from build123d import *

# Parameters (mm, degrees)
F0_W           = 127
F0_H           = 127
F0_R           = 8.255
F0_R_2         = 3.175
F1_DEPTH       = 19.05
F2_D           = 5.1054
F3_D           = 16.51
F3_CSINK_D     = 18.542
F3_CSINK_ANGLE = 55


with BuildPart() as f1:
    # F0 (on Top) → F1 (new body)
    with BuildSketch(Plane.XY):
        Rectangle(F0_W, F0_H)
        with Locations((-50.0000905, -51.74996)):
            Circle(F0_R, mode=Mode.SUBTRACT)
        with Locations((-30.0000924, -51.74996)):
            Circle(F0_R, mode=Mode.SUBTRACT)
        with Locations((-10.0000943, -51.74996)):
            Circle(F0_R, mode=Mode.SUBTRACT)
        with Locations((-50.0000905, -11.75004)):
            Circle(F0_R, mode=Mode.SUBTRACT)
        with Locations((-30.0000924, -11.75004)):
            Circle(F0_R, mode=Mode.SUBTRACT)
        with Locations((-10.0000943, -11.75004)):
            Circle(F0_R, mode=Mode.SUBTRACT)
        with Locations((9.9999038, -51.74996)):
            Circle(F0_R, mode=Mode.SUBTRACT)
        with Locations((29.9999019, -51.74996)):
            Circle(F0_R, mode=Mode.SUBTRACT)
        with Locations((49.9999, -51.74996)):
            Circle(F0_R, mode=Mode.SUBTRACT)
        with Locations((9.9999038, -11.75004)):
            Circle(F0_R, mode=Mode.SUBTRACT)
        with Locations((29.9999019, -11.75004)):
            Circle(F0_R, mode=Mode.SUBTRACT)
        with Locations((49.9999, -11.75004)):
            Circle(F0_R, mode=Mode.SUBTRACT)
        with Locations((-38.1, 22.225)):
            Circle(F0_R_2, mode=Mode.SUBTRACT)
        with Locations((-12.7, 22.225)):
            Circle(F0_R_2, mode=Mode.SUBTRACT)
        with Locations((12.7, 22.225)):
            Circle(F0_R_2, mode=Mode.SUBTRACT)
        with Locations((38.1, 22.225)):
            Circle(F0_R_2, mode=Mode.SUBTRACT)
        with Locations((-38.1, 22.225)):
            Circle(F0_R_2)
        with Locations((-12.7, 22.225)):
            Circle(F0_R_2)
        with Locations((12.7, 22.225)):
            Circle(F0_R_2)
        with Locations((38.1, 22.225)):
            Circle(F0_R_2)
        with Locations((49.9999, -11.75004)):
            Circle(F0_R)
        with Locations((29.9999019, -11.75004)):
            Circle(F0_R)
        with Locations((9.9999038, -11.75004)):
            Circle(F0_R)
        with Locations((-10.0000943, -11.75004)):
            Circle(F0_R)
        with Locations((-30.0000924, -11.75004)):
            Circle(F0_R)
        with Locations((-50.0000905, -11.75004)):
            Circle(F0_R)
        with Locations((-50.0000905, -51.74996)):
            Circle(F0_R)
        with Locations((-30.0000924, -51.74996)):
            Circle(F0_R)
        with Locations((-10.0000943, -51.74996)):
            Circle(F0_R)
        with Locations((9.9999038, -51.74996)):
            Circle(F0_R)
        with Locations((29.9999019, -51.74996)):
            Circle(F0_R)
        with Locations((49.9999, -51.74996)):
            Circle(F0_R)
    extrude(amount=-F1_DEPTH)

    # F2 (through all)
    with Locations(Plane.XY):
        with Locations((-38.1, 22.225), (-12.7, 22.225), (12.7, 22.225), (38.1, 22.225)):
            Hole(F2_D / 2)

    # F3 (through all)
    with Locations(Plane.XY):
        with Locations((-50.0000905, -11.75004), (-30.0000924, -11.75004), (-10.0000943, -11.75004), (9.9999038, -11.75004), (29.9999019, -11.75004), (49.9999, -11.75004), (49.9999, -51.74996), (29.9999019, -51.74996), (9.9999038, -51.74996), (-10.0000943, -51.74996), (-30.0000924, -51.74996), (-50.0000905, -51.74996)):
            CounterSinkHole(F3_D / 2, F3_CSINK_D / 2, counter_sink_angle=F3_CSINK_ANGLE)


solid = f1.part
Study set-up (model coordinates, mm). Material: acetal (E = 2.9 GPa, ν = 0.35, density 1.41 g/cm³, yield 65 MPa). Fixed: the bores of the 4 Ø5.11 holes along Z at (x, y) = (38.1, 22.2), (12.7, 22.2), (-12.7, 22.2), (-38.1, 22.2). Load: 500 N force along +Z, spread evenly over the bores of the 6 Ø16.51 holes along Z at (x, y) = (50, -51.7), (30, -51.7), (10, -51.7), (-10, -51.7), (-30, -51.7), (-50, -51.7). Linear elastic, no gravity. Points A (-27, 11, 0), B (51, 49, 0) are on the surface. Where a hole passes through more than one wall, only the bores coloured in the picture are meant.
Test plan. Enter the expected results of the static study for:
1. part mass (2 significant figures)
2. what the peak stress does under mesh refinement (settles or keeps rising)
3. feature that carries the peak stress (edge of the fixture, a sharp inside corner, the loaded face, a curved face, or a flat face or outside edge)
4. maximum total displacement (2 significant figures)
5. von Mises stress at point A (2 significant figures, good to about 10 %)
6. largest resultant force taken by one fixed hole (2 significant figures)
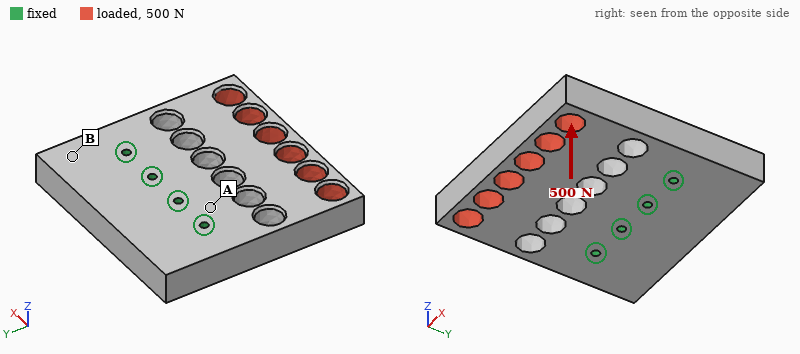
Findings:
360 g
keeps rising
edge of the fixture
0.77 mm
3.2 MPa
140 N
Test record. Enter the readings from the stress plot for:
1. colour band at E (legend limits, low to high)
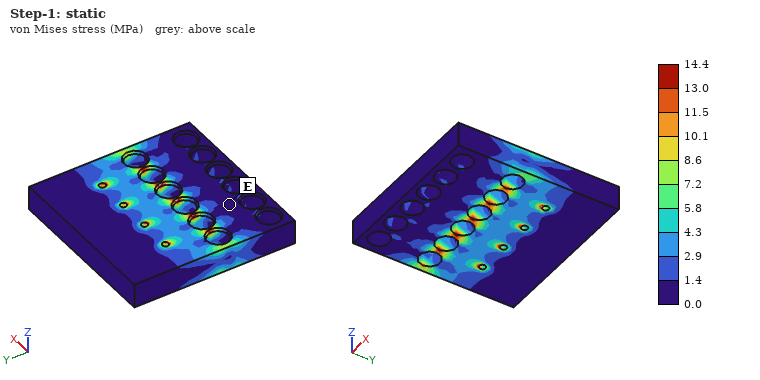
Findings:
0.0 to 1.4 MPa
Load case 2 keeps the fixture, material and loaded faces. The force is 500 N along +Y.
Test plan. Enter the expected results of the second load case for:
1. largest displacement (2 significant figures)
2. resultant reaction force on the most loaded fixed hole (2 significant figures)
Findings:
22 µm
160 N
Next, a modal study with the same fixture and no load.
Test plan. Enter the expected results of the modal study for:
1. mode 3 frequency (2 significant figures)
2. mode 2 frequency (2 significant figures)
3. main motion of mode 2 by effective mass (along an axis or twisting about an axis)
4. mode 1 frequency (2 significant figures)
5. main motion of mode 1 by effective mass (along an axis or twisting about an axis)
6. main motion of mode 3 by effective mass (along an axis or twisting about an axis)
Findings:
1300 Hz
840 Hz
twisting about Y
540 Hz
along Z
along X
